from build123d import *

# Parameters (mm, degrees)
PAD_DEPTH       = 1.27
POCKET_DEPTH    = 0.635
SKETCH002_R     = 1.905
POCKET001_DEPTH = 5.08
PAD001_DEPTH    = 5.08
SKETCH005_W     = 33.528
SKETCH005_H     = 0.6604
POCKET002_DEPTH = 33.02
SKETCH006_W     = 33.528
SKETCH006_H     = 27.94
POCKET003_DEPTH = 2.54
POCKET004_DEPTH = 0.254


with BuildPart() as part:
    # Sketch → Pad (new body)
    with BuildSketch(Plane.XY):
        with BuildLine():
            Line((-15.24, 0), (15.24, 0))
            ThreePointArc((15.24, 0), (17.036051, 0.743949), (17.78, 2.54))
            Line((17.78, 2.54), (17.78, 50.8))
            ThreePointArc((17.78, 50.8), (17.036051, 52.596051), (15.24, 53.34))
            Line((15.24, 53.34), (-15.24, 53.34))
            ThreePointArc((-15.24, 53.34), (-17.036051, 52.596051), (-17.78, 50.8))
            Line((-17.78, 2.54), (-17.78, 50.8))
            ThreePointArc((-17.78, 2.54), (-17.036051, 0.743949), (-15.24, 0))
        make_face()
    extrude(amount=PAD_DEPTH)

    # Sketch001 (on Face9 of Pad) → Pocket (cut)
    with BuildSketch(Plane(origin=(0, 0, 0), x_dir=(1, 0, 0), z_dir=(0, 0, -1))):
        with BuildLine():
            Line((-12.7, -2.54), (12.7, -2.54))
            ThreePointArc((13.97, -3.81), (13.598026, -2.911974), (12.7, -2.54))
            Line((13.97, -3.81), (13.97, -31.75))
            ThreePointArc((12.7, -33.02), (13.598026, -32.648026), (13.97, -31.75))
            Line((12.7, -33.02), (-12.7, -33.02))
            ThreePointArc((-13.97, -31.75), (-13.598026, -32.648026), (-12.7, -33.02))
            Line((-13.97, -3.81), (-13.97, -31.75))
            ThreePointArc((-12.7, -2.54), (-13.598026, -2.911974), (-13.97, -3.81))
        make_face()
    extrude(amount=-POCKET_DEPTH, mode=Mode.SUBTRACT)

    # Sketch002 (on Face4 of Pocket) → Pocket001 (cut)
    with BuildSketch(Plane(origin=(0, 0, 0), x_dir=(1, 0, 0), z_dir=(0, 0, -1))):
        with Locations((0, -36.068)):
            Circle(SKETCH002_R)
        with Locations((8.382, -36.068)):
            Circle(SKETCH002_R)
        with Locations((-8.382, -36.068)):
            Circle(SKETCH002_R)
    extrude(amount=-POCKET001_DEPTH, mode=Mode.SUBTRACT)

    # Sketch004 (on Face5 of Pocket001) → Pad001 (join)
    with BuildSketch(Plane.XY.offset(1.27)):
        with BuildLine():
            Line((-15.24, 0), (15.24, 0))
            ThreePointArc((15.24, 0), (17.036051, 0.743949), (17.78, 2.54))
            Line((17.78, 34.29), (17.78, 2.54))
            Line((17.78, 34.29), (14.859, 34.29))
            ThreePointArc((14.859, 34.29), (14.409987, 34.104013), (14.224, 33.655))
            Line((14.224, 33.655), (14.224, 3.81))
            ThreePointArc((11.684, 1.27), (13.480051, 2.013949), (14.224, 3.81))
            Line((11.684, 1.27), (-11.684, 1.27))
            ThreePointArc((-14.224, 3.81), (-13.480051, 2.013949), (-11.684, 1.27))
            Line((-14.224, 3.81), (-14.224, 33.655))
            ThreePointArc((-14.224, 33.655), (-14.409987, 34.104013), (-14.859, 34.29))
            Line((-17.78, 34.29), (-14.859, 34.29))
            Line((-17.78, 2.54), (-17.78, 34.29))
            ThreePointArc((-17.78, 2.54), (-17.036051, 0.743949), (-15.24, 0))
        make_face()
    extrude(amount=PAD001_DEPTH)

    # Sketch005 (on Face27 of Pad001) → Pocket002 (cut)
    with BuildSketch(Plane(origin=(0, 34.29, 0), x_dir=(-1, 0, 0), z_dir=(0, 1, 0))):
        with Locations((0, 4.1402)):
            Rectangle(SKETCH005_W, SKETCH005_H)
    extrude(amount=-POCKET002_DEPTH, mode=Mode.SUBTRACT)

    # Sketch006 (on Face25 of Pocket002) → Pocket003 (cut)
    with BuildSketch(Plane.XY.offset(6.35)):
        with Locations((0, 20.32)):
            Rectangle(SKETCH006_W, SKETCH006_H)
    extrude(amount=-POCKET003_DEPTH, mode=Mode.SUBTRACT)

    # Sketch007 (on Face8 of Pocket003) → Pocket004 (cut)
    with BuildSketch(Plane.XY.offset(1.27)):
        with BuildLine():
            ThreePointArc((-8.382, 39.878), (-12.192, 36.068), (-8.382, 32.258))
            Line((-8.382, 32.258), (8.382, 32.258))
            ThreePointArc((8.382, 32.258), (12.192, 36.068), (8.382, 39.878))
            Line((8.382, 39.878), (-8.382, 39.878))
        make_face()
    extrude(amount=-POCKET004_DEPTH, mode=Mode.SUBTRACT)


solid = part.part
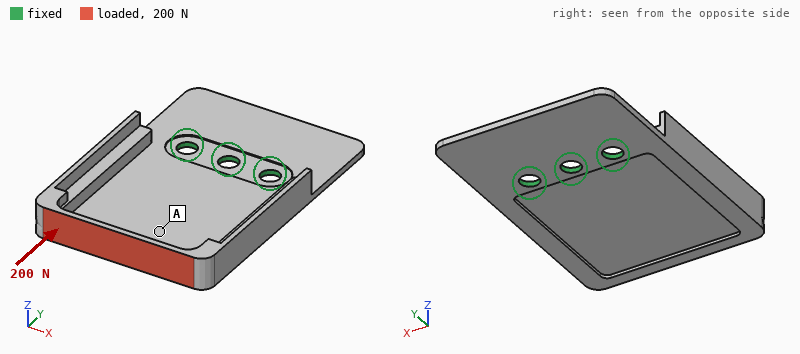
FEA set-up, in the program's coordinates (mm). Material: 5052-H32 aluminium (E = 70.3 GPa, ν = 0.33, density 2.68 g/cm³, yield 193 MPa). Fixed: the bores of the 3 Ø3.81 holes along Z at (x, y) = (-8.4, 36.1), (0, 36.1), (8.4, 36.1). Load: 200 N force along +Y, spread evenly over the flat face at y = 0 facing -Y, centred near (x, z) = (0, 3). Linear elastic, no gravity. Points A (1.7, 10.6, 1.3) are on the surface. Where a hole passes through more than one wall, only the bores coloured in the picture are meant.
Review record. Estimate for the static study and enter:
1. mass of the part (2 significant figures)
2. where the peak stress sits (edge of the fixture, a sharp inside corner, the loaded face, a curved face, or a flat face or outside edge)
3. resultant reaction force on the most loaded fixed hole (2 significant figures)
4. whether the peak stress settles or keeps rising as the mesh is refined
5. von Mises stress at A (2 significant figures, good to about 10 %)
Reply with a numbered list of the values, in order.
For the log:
1. 7.6 g
2. a sharp inside corner
3. 70 N
4. keeps rising
5. 14 MPa
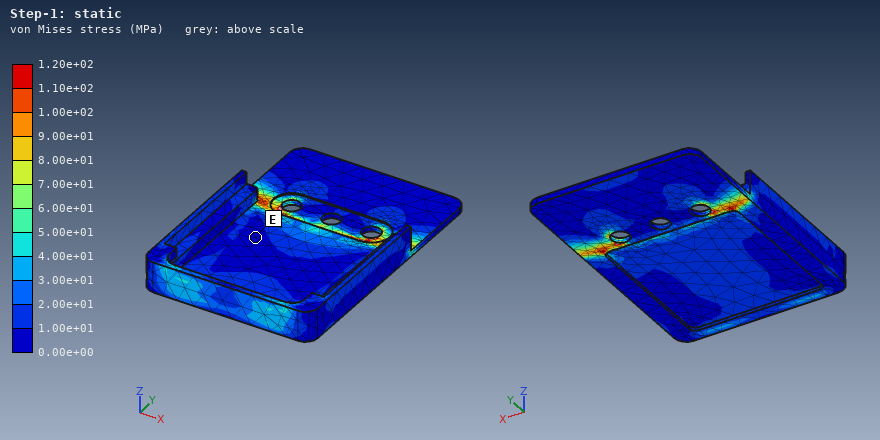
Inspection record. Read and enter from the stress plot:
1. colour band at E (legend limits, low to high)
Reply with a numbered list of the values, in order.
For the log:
1. 0.00e+00 to 1.00e+01 MPa
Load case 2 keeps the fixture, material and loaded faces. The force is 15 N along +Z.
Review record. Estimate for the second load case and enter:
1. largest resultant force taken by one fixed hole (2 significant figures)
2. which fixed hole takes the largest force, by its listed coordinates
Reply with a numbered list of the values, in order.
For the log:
1. 23 N
2. (0, 36.1)
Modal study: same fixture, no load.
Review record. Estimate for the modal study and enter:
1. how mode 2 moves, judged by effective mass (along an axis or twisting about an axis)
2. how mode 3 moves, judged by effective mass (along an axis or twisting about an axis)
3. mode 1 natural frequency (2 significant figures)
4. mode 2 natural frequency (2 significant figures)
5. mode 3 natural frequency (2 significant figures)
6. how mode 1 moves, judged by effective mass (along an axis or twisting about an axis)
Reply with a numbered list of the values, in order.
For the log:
1. twisting about Y
2. along Z
3. 610 Hz
4. 1300 Hz
5. 3500 Hz
6. along Z
